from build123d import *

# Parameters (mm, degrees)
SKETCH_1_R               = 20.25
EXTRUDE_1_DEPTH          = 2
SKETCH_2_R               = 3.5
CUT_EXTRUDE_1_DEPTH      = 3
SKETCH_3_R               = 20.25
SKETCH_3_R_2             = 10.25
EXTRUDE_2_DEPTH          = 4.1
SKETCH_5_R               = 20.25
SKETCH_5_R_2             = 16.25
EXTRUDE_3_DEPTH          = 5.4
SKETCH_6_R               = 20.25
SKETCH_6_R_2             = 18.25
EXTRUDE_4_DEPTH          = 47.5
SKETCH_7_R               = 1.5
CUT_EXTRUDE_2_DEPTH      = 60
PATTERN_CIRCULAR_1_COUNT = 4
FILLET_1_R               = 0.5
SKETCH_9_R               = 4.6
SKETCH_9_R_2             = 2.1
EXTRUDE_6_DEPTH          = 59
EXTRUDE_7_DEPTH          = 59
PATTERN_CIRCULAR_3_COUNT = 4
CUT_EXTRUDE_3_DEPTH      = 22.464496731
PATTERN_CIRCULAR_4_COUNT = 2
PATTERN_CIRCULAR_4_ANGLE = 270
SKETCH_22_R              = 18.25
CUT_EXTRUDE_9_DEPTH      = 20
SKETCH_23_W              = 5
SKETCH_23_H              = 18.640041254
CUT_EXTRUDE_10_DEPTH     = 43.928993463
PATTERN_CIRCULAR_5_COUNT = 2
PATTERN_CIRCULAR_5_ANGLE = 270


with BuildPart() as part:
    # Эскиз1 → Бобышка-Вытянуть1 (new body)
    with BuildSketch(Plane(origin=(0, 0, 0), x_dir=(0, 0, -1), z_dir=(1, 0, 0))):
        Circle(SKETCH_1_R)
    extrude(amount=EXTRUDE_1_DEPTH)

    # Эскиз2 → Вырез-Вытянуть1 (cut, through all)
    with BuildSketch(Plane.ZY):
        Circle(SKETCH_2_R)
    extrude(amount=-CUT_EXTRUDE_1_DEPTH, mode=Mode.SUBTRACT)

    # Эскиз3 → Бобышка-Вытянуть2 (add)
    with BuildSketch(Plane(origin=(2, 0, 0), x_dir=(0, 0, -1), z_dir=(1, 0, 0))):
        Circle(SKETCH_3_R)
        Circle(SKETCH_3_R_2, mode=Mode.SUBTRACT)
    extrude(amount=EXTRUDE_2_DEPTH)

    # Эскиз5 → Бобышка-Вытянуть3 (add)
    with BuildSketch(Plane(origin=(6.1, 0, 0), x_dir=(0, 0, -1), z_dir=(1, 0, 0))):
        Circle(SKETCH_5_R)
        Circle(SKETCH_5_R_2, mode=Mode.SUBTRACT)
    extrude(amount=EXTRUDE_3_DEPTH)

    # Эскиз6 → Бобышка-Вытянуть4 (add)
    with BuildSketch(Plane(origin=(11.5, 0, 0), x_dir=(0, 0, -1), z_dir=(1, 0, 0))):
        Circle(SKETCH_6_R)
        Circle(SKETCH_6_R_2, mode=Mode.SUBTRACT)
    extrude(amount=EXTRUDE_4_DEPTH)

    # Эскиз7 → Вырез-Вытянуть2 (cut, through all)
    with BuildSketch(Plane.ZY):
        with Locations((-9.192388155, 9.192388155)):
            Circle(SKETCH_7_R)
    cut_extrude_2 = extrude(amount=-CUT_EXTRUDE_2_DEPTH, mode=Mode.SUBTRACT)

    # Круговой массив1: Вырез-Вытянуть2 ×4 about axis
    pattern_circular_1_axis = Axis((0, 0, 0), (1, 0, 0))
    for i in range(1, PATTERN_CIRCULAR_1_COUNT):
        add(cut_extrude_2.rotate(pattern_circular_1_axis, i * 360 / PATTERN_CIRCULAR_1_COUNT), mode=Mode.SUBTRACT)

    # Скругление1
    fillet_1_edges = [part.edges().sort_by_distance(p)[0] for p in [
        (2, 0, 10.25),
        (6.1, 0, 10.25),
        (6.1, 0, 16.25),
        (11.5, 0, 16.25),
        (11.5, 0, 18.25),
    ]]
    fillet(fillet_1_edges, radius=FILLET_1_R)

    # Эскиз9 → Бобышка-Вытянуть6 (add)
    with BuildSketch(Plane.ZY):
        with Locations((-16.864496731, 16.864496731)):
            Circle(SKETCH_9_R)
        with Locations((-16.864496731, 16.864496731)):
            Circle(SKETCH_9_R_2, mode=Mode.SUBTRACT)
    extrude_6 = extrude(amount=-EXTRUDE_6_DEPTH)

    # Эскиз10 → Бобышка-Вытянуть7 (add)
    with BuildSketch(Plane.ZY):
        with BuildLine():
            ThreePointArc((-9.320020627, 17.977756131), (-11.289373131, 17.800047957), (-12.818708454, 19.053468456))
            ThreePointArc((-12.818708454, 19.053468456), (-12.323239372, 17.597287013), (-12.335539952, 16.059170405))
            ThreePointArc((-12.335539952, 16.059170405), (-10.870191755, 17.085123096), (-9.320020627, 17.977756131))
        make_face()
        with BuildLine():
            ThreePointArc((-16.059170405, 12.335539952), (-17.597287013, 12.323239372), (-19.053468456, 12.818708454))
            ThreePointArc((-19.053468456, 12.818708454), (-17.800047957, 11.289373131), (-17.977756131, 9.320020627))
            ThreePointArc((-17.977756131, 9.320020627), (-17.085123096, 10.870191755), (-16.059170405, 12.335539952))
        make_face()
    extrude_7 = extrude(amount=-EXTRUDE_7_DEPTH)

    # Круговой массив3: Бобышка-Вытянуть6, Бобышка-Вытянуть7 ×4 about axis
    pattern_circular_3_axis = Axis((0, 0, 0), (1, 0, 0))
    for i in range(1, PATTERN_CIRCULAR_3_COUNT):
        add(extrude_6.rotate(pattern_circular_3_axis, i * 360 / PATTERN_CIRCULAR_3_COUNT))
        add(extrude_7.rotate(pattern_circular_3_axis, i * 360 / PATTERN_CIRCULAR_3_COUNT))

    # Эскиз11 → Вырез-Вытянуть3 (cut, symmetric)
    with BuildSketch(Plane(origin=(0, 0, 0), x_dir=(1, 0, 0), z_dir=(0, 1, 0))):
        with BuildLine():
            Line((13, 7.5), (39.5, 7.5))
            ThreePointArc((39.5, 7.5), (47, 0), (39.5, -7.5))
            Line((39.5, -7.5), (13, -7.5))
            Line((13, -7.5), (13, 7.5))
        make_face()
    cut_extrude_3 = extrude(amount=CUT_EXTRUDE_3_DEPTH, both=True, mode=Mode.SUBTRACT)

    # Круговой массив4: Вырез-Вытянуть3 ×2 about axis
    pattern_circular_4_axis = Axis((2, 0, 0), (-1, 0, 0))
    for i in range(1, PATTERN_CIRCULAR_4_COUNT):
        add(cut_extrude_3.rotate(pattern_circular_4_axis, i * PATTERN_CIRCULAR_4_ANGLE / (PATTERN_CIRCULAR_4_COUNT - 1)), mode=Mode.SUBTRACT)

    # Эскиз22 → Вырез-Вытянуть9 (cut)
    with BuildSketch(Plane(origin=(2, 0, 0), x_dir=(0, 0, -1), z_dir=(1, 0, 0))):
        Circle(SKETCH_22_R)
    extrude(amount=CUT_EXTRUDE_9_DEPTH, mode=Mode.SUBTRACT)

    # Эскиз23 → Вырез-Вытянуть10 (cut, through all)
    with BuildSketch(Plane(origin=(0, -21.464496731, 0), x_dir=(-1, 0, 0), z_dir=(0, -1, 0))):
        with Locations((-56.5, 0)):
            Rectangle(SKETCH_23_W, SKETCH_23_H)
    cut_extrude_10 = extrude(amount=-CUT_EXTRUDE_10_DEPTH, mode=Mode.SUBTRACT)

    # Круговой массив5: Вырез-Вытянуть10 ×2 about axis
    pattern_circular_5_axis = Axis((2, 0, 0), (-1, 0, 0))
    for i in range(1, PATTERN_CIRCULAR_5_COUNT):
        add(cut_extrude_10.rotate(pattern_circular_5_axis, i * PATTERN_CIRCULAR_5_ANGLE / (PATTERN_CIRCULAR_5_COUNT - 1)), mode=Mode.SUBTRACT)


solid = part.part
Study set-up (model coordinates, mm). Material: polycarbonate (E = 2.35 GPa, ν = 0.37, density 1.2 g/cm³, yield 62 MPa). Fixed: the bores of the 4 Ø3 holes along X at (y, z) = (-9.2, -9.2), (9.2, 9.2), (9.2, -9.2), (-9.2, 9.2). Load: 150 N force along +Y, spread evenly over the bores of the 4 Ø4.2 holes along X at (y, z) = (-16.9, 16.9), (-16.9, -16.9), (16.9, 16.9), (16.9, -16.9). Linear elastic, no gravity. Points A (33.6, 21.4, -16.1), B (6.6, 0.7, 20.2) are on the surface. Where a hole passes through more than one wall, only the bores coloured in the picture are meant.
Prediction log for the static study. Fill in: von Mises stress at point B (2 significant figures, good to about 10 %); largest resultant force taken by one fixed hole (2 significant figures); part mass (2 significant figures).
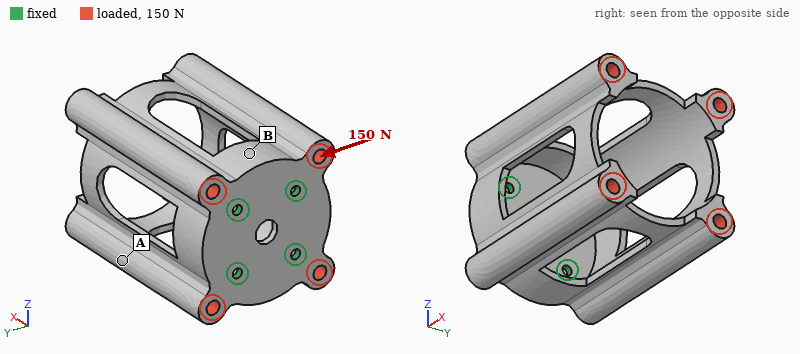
4.7 MPa
100 N
29 g
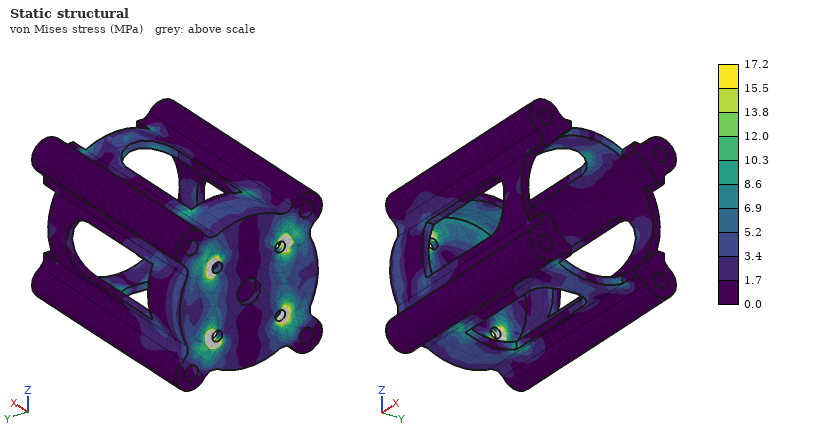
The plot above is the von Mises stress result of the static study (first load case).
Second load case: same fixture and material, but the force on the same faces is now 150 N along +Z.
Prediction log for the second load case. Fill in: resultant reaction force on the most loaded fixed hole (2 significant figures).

100 N
